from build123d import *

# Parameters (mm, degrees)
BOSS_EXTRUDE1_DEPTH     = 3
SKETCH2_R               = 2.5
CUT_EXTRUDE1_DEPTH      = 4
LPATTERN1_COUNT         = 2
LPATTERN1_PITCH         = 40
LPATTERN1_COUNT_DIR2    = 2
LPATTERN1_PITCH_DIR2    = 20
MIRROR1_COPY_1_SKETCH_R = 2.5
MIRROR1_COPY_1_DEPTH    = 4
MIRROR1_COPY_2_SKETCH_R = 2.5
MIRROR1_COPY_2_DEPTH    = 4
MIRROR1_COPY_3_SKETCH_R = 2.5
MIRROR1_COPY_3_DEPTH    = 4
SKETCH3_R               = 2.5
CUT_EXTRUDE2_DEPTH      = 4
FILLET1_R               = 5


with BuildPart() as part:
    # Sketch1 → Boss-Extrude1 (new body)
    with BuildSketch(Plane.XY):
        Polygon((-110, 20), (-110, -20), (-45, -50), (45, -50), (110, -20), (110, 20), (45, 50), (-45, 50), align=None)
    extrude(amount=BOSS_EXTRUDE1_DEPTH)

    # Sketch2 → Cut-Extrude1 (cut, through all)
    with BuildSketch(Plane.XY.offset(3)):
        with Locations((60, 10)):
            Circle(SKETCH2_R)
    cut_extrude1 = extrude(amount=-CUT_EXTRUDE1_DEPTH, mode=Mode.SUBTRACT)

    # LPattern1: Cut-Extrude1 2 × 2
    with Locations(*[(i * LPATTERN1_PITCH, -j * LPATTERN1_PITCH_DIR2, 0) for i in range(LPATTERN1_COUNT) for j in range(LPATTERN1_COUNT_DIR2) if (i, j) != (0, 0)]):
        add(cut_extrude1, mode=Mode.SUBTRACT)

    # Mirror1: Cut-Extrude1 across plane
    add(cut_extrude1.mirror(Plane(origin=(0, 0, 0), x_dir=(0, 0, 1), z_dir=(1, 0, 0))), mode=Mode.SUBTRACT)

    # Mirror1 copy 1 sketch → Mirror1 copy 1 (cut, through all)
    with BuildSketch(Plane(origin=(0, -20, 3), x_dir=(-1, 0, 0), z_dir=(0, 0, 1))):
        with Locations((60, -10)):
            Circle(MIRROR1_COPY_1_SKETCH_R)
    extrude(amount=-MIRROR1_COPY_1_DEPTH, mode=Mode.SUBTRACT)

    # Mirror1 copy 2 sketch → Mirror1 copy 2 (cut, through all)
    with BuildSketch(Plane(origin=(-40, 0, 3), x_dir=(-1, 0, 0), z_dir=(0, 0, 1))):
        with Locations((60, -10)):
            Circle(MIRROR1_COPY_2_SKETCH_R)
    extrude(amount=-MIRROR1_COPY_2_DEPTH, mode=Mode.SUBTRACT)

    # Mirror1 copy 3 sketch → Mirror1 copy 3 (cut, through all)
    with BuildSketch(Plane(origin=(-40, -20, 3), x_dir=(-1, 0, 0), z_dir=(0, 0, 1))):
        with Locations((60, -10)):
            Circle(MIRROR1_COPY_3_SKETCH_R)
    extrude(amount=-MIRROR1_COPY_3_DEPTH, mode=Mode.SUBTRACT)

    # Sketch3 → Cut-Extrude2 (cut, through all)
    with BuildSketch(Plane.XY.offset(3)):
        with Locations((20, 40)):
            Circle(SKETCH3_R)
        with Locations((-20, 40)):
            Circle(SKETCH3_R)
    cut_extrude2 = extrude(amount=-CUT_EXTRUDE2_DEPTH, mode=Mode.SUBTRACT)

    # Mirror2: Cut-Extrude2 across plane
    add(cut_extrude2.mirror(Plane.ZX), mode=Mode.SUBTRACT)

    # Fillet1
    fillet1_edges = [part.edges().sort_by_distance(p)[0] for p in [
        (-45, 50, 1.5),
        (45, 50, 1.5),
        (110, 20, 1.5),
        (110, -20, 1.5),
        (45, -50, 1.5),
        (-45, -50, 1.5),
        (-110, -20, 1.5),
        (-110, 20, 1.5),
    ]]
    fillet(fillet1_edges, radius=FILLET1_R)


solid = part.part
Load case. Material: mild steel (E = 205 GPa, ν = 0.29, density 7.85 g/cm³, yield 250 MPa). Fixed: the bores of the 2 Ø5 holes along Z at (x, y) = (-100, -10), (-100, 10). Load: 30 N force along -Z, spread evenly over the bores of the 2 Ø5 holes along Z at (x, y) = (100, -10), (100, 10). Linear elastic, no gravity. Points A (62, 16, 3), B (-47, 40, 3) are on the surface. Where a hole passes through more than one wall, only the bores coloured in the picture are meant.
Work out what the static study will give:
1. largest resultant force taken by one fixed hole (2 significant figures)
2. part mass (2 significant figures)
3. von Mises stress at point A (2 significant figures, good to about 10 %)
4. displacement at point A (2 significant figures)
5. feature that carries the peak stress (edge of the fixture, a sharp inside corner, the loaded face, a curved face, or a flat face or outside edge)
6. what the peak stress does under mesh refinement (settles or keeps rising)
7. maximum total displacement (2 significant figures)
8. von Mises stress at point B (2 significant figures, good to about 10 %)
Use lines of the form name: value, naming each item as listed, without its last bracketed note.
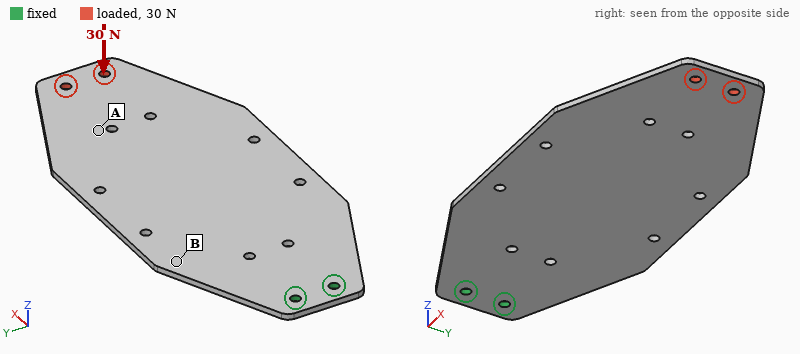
largest resultant force taken by one fixed hole: 15 N
part mass: 420 g
von Mises stress at point A: 11 MPa
displacement at point A: 1.6 mm
feature that carries the peak stress: edge of the fixture
what the peak stress does under mesh refinement: keeps rising
maximum total displacement: 2.4 mm
von Mises stress at point B: 28 MPa
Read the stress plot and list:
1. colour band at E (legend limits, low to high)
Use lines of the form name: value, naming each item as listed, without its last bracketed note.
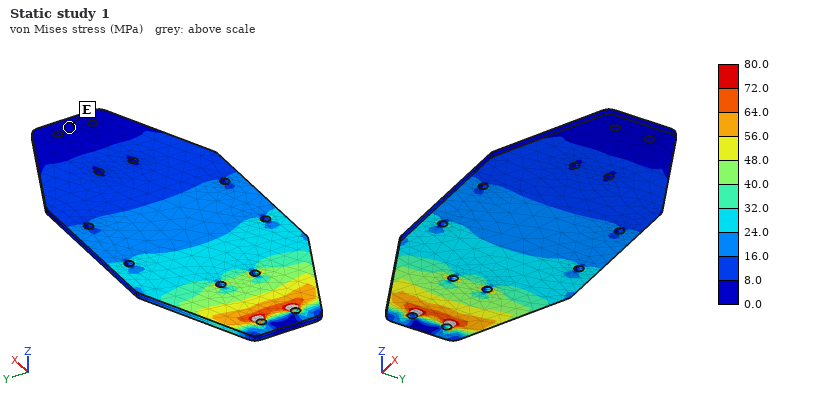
colour band at E: 0.0 to 8.0 MPa
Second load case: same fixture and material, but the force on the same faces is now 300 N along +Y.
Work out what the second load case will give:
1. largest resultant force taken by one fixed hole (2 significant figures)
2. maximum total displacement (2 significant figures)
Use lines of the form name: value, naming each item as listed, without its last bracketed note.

largest resultant force taken by one fixed hole: 2.5 kN
maximum total displacement: 0.10 mm
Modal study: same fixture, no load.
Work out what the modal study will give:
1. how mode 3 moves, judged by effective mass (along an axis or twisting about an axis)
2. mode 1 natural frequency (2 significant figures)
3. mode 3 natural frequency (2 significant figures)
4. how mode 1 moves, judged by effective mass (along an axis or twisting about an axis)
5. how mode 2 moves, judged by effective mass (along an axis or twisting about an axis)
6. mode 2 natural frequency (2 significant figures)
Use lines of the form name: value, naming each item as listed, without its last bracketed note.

how mode 3 moves, judged by effective mass: along Z
mode 1 natural frequency: 57 Hz
mode 3 natural frequency: 360 Hz
how mode 1 moves, judged by effective mass: along Z
how mode 2 moves, judged by effective mass: twisting about X
mode 2 natural frequency: 260 Hz
